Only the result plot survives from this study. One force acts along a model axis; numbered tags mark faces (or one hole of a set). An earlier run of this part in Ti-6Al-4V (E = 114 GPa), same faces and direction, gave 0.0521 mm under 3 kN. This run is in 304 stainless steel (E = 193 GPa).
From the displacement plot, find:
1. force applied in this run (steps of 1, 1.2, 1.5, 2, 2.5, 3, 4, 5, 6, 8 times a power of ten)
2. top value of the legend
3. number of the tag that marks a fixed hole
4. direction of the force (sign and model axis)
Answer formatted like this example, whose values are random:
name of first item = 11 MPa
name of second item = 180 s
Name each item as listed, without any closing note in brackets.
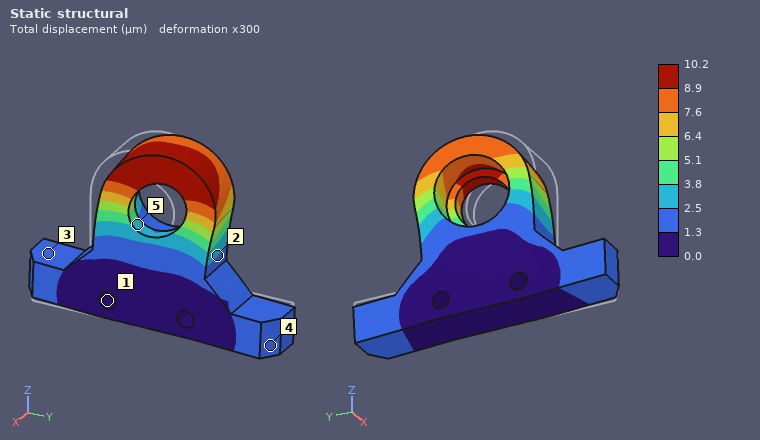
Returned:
force applied in this run = 1 kN
top value of the legend = 10.2 µm
number of the tag that marks a fixed hole = 1
direction of the force = +Y
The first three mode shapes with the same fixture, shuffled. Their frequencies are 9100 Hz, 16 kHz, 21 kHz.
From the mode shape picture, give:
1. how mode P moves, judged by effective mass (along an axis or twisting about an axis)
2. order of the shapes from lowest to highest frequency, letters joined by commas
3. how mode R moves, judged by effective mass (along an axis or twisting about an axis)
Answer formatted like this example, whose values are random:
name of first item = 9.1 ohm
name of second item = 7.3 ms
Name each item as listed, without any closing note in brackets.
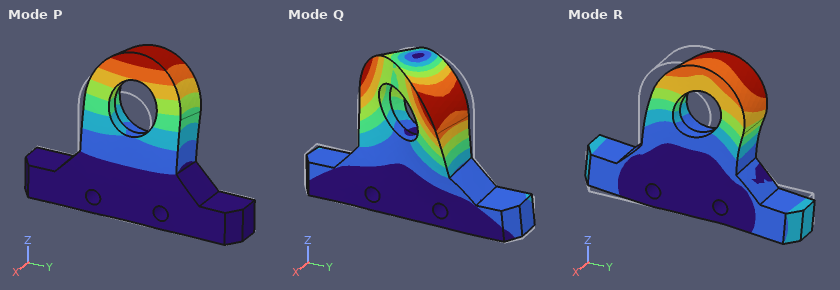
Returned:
how mode P moves, judged by effective mass = along X
order of the shapes from lowest to highest frequency, letters joined by commas = P, R, Q
how mode R moves, judged by effective mass = along Y
